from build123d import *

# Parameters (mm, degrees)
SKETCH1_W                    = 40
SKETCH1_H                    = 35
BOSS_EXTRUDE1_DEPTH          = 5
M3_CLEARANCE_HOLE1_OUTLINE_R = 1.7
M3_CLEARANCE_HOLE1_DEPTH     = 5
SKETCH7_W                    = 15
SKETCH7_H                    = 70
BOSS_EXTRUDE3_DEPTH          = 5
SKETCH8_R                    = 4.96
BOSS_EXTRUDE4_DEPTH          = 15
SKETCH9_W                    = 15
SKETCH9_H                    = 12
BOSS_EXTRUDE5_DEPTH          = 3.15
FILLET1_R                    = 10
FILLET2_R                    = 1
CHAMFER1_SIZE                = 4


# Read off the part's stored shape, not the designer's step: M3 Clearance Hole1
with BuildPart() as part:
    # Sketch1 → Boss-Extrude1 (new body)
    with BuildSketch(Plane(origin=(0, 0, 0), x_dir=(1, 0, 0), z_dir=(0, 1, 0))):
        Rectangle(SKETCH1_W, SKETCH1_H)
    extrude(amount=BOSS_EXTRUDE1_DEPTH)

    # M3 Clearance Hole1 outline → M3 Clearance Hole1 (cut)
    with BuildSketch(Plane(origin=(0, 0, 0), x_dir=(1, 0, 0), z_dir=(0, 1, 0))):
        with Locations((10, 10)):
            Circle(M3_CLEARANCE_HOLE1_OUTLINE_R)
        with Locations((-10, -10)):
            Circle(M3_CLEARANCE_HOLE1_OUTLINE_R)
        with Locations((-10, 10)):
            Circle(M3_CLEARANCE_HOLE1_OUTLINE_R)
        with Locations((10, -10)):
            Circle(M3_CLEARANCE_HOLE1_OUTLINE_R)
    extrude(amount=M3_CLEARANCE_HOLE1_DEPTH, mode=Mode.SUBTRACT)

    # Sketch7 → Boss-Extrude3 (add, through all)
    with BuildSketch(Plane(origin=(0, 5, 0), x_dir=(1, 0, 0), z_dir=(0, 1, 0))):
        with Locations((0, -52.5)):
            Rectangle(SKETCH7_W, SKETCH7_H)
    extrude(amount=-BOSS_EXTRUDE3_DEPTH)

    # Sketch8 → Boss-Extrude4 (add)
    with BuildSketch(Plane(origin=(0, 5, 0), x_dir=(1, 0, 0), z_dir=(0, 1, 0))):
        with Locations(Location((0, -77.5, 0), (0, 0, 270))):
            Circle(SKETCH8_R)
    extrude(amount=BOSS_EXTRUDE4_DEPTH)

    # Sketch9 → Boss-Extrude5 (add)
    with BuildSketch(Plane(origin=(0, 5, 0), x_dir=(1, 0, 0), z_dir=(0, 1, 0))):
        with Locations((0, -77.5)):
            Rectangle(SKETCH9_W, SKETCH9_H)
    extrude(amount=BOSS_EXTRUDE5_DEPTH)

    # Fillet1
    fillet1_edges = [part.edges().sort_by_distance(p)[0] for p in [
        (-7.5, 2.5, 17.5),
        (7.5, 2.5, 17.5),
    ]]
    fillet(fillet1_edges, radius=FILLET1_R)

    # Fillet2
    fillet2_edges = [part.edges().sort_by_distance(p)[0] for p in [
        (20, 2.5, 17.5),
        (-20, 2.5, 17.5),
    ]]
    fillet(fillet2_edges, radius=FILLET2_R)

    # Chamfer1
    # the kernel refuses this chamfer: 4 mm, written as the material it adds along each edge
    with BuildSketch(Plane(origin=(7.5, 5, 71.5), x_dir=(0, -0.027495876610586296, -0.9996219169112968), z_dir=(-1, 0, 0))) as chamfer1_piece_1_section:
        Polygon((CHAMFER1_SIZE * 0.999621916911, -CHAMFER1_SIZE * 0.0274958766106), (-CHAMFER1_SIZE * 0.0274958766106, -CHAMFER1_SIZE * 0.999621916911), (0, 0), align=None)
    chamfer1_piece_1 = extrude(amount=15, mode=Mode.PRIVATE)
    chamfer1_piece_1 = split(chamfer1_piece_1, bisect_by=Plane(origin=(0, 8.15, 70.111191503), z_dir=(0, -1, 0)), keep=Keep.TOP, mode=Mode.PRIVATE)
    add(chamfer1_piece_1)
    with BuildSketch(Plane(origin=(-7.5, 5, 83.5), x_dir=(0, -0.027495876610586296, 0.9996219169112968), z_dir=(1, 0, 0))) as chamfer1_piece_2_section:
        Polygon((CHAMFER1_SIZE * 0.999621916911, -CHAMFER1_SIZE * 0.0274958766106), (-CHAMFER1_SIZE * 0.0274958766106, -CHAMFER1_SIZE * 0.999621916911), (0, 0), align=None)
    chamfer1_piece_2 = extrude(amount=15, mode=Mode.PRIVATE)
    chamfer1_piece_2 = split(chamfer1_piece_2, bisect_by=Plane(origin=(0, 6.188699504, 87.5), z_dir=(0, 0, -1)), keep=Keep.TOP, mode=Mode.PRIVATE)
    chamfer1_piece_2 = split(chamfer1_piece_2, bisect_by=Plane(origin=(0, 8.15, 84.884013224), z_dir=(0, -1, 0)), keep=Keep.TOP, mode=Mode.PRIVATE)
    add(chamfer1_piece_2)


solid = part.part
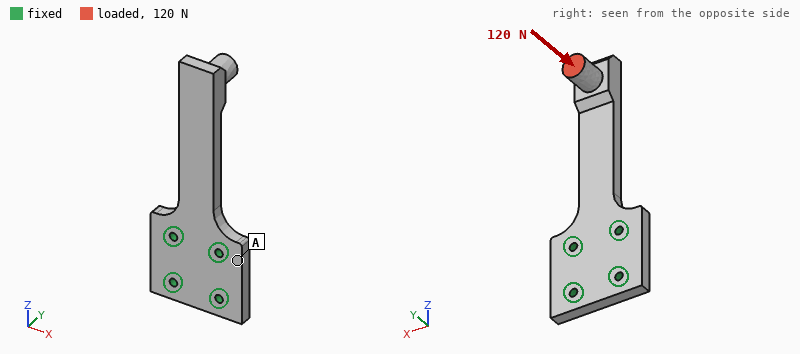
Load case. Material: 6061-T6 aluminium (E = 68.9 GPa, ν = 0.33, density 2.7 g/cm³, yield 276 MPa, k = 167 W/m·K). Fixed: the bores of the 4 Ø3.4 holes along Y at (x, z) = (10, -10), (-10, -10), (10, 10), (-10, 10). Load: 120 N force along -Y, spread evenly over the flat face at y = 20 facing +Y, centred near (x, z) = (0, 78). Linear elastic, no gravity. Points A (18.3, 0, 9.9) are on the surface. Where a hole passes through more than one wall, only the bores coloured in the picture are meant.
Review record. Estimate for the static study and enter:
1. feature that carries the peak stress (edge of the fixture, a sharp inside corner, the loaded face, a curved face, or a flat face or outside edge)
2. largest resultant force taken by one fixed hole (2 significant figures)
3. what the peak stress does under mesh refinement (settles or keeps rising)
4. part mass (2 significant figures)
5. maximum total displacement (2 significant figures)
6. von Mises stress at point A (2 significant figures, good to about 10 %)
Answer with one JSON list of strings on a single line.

["edge of the fixture", "120 N", "keeps rising", "38 g", "1.2 mm", "12 MPa"]
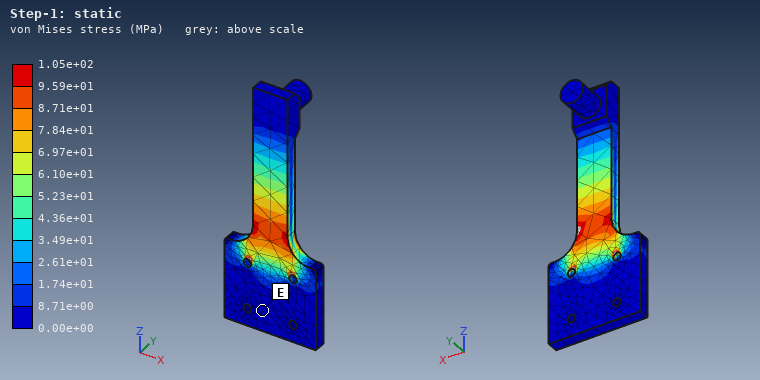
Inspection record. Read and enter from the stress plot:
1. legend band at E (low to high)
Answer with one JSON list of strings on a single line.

["0.00e+00 to 8.71e+00 MPa"]
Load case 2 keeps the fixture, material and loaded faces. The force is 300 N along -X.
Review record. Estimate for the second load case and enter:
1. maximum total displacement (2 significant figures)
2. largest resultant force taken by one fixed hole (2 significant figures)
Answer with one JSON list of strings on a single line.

["0.60 mm", "870 N"]
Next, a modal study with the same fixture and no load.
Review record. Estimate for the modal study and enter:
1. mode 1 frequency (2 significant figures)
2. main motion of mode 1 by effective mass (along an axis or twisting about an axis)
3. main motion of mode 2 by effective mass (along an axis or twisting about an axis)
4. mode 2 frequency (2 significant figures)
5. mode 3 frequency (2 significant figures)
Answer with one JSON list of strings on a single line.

["550 Hz", "along Y", "along X", "1800 Hz", "3800 Hz"]
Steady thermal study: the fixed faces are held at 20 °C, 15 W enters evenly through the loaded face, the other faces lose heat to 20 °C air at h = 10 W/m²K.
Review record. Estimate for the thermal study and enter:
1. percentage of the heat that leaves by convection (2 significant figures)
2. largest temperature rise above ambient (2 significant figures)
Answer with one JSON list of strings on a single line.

["10 %", "81 K"]
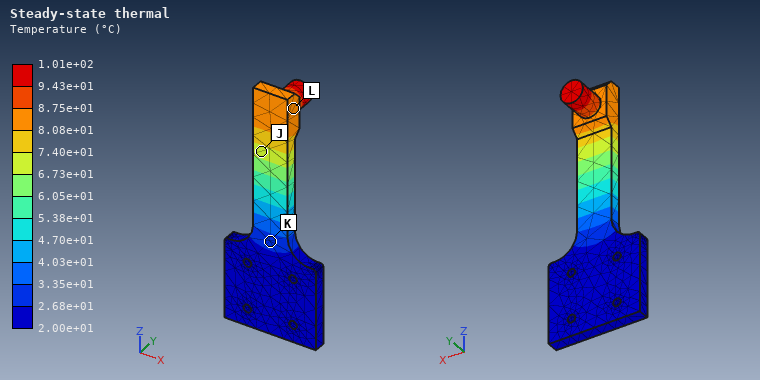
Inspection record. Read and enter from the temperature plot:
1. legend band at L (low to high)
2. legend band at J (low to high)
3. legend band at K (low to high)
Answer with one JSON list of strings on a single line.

["8.08e+01 to 8.75e+01 °C", "6.73e+01 to 7.40e+01 °C", "2.68e+01 to 3.35e+01 °C"]
